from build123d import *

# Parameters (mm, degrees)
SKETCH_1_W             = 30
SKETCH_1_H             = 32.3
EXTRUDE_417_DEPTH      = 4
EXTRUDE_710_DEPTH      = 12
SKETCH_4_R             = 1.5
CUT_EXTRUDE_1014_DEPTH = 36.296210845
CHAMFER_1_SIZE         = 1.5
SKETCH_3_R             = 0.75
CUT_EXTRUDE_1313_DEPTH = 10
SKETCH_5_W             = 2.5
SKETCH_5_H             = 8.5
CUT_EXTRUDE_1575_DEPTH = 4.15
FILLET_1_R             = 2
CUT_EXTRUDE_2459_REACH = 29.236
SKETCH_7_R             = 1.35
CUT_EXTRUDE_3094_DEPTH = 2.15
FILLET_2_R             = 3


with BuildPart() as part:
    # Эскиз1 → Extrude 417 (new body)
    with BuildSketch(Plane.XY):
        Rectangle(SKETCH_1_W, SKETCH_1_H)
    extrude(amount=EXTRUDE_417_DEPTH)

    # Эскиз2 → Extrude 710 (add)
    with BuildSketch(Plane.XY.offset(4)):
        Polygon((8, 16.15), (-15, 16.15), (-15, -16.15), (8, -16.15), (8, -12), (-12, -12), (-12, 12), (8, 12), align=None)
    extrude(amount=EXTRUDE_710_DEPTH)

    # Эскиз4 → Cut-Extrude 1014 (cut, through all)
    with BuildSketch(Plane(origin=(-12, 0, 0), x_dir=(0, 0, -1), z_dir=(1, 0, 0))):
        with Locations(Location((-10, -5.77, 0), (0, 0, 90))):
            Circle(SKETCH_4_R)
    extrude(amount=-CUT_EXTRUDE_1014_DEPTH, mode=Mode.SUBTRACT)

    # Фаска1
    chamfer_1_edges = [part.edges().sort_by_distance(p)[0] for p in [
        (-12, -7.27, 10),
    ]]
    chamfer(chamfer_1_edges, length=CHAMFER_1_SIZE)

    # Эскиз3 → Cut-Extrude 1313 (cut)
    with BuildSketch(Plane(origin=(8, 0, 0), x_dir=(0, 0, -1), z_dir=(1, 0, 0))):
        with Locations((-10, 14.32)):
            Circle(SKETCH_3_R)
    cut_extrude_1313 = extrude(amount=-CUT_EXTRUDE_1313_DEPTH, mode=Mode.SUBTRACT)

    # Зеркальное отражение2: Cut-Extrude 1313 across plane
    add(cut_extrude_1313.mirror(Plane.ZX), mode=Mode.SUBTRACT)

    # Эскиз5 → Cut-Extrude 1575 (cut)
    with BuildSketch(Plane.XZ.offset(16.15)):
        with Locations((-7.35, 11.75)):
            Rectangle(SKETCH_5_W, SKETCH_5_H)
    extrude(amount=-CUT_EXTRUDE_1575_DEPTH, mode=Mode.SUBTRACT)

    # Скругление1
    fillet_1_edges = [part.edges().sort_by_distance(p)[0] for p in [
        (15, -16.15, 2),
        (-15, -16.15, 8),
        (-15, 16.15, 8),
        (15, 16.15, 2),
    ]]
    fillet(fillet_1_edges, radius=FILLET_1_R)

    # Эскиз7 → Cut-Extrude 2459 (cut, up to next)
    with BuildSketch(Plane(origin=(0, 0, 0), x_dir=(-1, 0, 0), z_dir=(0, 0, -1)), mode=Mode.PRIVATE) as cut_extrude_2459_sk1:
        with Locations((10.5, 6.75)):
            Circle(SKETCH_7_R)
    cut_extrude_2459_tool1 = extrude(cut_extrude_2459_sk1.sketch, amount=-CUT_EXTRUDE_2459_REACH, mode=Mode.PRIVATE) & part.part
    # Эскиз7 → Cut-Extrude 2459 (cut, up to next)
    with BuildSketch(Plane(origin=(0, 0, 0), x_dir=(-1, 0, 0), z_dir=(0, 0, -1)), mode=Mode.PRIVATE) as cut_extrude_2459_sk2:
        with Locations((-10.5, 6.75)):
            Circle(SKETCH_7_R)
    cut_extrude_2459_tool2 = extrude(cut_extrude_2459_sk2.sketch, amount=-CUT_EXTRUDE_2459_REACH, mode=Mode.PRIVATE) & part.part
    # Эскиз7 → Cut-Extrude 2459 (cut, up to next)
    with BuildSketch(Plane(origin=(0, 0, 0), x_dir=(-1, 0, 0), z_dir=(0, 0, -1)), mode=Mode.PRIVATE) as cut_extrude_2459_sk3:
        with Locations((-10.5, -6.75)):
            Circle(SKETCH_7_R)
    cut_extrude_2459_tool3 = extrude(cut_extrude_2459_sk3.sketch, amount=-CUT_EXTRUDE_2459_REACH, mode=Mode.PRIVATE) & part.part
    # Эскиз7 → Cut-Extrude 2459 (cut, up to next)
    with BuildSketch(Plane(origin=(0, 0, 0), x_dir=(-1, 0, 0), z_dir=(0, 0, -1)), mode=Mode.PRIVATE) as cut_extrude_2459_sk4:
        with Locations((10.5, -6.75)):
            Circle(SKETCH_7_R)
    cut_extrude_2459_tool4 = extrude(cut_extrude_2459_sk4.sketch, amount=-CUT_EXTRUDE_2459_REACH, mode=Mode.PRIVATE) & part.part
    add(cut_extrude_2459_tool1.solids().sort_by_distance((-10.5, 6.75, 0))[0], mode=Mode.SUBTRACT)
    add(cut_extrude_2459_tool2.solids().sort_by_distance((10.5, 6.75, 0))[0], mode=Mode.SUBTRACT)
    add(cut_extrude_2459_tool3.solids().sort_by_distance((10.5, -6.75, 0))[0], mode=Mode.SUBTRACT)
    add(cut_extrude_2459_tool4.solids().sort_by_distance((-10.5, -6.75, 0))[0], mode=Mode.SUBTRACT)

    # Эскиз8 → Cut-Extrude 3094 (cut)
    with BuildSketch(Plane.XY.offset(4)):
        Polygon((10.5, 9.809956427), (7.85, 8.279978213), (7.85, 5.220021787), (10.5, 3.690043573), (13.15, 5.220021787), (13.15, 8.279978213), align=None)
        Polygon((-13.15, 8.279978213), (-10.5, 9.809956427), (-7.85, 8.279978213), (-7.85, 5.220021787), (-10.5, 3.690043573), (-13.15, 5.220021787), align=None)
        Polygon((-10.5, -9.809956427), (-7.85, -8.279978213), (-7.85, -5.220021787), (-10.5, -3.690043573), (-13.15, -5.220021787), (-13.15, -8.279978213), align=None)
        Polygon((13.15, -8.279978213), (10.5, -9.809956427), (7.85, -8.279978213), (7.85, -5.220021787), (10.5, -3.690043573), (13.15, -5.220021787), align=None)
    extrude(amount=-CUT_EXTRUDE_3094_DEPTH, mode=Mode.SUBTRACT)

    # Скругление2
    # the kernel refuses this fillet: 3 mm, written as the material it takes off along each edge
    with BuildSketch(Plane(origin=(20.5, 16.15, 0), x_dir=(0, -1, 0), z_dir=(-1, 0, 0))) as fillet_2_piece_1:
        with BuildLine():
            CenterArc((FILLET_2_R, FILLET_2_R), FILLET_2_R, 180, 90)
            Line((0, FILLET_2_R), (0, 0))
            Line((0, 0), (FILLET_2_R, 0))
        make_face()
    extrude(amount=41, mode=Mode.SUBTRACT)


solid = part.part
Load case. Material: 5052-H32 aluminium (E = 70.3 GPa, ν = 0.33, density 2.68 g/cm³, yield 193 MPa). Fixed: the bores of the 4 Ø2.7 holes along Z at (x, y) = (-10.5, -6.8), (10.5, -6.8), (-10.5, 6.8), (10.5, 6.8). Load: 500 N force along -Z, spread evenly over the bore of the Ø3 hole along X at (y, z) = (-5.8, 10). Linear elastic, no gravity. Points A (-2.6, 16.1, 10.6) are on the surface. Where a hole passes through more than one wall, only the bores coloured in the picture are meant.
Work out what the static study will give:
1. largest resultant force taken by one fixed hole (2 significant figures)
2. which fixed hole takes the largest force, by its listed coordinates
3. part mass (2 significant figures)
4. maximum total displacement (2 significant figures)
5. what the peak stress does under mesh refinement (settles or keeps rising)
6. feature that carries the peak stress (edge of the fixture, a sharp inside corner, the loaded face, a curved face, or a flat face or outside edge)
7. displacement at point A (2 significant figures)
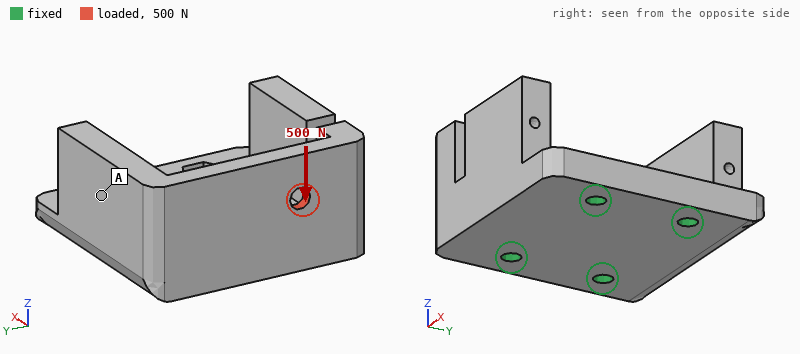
480 N
(-10.5, -6.8)
18 g
14 µm
keeps rising
edge of the fixture
3.3 µm
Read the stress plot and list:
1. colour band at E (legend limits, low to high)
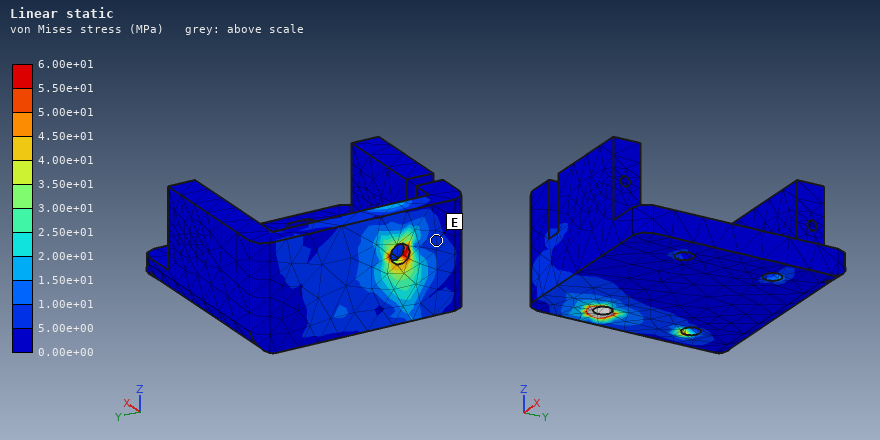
5.00e+00 to 1.00e+01 MPa
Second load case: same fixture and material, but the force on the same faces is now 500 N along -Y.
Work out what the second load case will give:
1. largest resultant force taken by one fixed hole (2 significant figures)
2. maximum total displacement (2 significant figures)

380 N
13 µm
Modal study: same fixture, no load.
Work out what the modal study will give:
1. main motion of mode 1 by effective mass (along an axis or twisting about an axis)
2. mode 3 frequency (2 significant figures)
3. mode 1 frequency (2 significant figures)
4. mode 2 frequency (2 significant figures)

along Y
15 kHz
10 kHz
12 kHz
